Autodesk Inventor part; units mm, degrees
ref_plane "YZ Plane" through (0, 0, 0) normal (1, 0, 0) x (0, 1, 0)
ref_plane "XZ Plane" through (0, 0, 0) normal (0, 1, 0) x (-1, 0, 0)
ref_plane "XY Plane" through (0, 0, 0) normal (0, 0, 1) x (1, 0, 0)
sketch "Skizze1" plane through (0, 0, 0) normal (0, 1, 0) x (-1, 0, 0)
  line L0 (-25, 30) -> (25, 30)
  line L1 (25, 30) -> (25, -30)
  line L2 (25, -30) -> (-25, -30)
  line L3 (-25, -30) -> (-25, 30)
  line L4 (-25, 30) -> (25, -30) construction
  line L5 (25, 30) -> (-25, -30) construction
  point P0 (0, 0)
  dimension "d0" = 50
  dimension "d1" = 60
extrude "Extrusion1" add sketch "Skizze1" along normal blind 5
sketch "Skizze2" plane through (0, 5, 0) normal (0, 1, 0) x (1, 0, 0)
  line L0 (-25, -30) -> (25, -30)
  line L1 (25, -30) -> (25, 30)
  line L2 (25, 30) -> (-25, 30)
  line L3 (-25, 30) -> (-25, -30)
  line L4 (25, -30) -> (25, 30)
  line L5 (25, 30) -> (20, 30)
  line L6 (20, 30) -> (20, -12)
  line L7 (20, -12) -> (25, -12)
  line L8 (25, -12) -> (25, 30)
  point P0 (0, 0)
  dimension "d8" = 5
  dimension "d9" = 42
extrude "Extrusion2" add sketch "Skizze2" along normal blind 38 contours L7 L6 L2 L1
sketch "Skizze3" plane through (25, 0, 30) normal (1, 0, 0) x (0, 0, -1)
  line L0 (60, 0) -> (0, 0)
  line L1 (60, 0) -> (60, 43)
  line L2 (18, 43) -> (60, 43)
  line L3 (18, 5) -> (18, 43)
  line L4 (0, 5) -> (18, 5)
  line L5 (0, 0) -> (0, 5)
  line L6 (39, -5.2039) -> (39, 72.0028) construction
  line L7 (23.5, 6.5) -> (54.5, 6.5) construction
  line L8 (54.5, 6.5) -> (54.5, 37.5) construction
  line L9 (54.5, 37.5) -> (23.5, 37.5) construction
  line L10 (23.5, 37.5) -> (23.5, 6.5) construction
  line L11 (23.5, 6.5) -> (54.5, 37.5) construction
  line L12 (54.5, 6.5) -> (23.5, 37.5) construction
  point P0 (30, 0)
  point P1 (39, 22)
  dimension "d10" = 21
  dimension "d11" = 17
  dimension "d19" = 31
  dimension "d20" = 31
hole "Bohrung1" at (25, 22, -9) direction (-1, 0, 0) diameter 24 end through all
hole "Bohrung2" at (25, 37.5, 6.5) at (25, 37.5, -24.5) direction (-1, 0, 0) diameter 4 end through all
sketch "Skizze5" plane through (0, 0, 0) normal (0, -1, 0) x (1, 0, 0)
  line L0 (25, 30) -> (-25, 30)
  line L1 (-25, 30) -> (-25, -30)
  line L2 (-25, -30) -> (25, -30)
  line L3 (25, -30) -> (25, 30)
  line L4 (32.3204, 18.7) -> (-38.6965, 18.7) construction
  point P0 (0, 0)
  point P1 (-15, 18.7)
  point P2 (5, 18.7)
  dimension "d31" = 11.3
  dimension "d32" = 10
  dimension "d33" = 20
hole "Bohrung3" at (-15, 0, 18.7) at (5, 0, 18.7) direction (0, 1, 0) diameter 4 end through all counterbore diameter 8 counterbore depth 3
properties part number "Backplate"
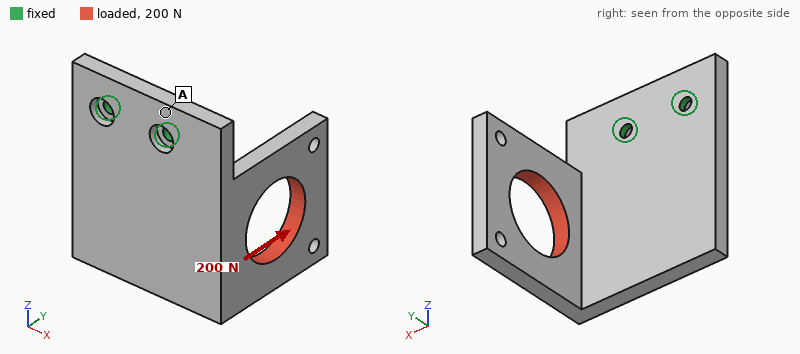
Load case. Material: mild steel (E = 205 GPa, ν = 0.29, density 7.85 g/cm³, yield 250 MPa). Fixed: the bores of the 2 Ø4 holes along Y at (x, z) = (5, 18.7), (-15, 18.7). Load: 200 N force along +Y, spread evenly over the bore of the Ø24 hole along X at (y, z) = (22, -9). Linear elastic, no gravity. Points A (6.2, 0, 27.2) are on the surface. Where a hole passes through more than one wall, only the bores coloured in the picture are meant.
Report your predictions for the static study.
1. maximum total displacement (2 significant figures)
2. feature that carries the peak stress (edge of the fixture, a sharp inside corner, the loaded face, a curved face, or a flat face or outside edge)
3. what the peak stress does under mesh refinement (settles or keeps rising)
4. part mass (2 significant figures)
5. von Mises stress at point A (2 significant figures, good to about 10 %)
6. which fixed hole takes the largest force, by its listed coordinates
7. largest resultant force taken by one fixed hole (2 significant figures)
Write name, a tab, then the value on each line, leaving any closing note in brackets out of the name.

maximum total displacement	0.13 mm
feature that carries the peak stress	edge of the fixture
what the peak stress does under mesh refinement	keeps rising
part mass	160 g
von Mises stress at point A	14 MPa
which fixed hole takes the largest force, by its listed coordinates	(5, 18.7)
largest resultant force taken by one fixed hole	350 N
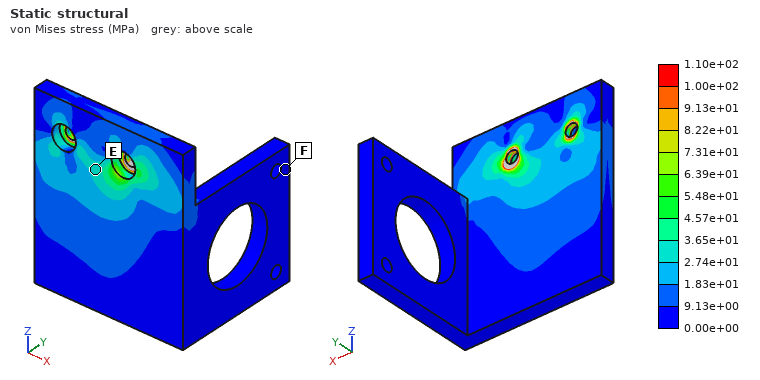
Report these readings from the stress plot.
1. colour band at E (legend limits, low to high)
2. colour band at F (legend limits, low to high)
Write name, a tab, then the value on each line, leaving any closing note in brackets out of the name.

colour band at E	2.74e+01 to 3.65e+01 MPa
colour band at F	0.00e+00 to 9.13e+00 MPa
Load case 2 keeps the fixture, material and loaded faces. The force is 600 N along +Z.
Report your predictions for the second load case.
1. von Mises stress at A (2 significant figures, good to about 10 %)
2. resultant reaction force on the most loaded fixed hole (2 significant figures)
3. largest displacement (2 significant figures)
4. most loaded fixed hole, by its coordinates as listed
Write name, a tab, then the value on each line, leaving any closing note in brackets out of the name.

von Mises stress at A	49 MPa
resultant reaction force on the most loaded fixed hole	1.1 kN
largest displacement	0.27 mm
most loaded fixed hole, by its coordinates as listed	(5, 18.7)
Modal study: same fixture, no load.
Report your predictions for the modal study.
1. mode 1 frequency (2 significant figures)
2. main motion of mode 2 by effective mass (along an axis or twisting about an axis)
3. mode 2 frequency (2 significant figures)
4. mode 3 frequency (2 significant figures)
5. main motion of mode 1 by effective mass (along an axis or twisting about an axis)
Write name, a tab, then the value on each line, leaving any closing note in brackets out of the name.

mode 1 frequency	760 Hz
main motion of mode 2 by effective mass	along X
mode 2 frequency	1300 Hz
mode 3 frequency	3100 Hz
main motion of mode 1 by effective mass	along Y
